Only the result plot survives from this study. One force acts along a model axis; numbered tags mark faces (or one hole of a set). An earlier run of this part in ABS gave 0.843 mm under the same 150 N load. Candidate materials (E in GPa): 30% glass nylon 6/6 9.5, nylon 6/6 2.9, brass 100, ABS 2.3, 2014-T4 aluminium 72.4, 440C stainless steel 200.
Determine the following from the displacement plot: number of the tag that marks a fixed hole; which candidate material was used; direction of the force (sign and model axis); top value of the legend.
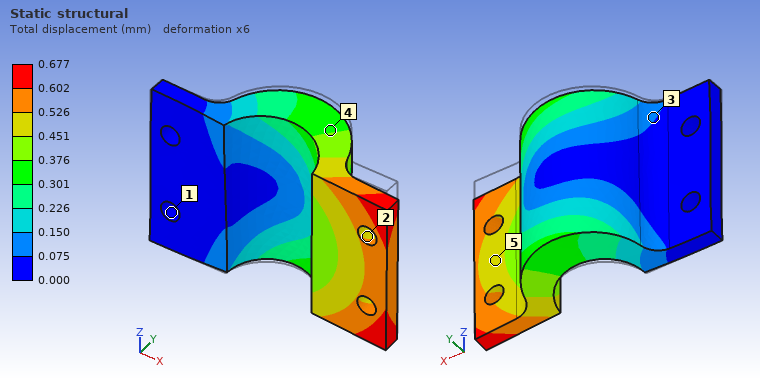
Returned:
1
nylon 6/6
-Z
0.677 mm
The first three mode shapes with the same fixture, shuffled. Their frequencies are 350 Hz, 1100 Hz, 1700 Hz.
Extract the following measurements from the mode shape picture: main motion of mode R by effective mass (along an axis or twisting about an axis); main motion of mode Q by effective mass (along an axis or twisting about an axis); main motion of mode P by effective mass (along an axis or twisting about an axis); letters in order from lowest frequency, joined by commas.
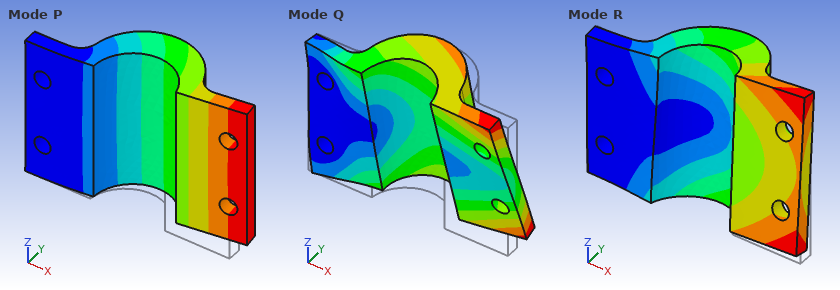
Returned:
along Z
along Z
along Y
P, R, Q
